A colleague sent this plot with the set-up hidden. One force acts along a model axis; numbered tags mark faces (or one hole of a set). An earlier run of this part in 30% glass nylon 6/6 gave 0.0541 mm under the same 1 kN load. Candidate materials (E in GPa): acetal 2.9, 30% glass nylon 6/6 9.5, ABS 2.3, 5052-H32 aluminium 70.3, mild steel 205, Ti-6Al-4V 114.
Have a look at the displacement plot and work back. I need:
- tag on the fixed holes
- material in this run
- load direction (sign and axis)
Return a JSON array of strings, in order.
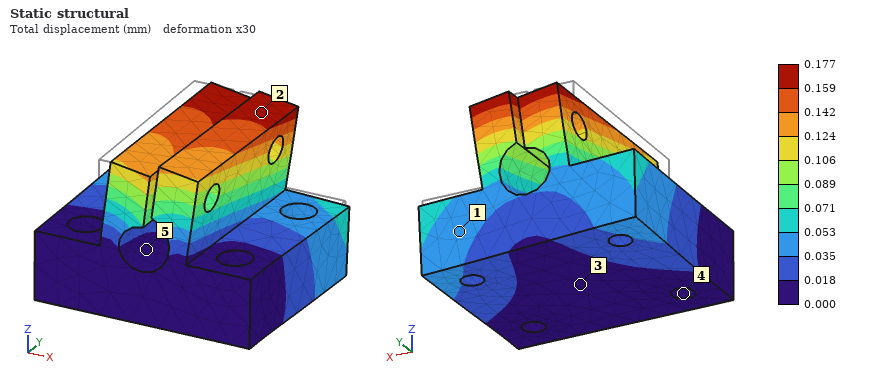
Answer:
["4", "acetal", "+X"]
